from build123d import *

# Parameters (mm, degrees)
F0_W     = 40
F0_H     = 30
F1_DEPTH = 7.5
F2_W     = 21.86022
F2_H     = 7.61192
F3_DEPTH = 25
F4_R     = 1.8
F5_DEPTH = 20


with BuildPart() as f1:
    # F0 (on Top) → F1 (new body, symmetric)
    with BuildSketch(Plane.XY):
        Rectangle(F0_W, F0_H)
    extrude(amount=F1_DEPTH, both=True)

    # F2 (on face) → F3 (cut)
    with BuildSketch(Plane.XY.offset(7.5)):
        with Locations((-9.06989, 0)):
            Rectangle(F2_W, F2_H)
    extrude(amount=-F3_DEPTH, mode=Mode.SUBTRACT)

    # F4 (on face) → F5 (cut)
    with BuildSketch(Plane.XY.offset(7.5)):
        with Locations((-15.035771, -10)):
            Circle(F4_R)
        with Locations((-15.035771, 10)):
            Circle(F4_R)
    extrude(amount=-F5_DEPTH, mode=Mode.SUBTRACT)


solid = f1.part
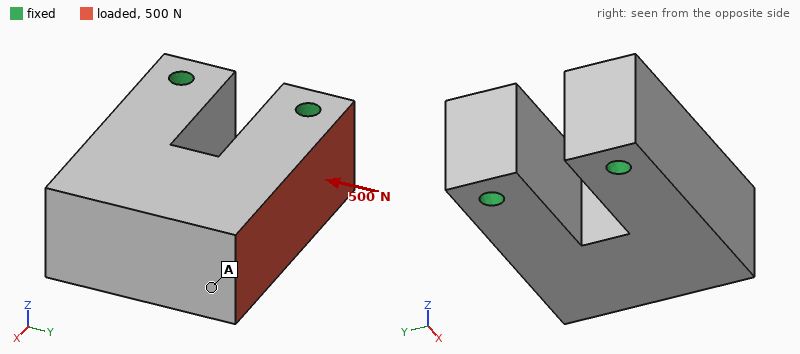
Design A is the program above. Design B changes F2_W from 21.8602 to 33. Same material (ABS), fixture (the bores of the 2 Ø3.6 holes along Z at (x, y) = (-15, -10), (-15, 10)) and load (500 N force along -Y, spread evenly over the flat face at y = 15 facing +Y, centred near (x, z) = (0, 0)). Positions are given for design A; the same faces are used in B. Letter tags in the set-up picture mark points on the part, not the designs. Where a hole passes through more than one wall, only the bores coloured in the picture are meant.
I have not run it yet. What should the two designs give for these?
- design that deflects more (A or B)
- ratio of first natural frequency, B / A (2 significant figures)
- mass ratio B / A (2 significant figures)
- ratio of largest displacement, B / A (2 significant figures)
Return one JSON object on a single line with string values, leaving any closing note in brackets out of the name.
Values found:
{"design that deflects more": "B", "ratio of first natural frequency, B / A": "1.0", "mass ratio B / A": "0.96", "ratio of largest displacement, B / A": "1.3"}
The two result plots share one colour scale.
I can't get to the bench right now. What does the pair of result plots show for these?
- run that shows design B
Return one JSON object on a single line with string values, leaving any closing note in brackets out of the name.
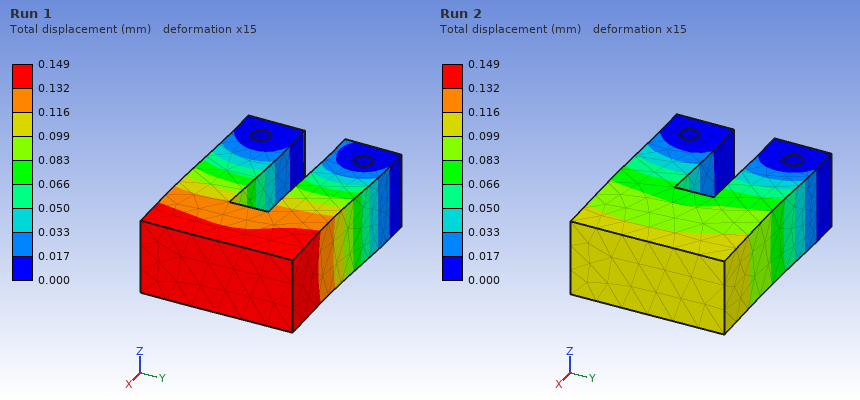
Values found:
{"run that shows design B": "Run 1"}
